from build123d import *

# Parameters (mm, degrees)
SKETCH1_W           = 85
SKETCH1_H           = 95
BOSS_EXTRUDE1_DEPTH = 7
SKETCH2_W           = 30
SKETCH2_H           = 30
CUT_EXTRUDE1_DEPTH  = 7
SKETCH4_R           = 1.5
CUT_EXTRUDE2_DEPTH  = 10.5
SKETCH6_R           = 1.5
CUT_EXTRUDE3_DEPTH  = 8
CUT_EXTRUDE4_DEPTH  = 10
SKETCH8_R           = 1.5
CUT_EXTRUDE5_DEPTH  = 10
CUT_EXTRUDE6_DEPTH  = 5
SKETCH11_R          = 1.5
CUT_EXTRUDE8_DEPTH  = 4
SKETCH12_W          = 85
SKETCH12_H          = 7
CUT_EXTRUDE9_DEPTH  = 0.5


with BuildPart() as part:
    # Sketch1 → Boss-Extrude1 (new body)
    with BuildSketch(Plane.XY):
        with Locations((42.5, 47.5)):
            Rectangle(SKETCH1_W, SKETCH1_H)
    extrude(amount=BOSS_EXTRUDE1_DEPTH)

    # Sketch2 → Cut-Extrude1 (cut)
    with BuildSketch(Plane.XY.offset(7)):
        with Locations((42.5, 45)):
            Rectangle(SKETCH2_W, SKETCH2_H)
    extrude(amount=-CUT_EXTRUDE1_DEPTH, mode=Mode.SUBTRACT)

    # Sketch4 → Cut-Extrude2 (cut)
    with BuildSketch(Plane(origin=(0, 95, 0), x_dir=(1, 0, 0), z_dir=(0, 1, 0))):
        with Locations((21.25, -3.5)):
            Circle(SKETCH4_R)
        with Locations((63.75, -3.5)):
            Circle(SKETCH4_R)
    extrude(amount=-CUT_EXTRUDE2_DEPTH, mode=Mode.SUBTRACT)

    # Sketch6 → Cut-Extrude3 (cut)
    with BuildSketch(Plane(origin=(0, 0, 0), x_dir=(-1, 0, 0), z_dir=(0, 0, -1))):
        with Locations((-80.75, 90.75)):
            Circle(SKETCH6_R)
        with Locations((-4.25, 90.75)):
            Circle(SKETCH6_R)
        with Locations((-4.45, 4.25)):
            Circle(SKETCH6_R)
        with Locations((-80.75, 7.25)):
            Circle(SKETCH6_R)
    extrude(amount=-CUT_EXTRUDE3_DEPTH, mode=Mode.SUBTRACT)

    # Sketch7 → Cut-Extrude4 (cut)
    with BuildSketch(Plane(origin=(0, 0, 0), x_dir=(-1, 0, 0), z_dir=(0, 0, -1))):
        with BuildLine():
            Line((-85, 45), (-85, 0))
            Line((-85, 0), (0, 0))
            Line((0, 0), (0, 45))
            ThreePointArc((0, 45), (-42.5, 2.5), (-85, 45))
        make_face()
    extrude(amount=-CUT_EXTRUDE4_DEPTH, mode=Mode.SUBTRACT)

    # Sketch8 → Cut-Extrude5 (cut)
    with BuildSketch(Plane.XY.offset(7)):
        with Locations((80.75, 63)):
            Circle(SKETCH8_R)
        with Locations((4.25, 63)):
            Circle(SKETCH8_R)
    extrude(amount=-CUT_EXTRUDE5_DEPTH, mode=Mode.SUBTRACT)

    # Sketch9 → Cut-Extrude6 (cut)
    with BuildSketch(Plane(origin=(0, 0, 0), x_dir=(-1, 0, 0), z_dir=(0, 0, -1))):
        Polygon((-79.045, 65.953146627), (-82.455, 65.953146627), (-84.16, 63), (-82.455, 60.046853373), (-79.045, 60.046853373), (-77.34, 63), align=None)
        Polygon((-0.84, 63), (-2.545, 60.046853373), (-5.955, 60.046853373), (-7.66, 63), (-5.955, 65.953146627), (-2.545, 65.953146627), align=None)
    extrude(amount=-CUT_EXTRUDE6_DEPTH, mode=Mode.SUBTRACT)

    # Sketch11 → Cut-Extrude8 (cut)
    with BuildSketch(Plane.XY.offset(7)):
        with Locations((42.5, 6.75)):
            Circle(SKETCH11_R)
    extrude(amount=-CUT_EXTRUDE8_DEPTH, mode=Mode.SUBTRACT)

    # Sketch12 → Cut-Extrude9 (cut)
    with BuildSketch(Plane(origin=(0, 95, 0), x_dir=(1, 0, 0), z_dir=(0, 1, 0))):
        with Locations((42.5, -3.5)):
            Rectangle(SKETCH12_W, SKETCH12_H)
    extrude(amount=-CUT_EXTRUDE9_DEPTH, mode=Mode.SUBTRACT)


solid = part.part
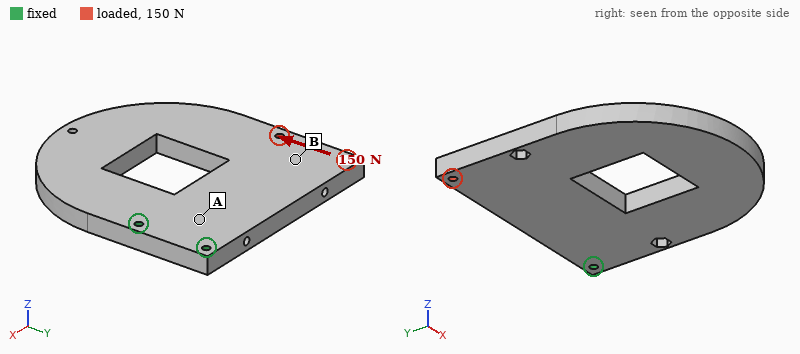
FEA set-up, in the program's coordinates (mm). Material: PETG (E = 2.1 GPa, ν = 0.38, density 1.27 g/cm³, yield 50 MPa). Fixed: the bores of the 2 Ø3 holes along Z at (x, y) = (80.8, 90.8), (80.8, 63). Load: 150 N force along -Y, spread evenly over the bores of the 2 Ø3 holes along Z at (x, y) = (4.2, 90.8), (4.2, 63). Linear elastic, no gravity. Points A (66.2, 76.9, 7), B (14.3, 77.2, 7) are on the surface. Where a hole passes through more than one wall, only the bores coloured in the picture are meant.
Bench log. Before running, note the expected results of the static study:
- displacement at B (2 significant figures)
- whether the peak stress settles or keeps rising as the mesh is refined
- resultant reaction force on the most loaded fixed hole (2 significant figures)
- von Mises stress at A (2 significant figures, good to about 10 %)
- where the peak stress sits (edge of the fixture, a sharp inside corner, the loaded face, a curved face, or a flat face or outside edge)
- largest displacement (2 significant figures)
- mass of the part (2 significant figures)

0.82 mm
keeps rising
410 N
3.7 MPa
edge of the fixture
1.3 mm
54 g
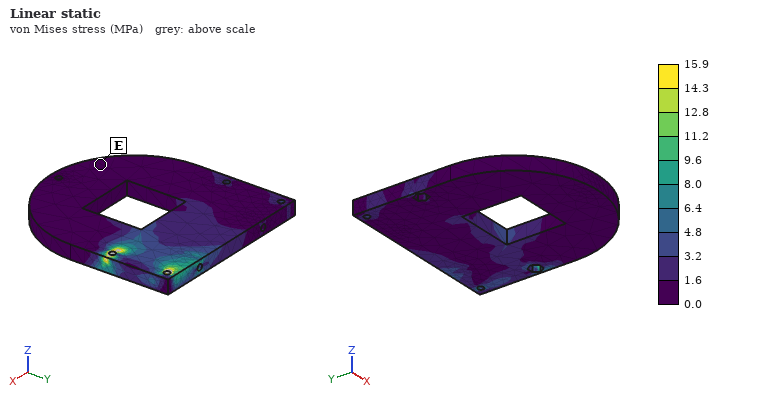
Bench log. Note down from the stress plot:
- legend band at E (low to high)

0.0 to 1.6 MPa
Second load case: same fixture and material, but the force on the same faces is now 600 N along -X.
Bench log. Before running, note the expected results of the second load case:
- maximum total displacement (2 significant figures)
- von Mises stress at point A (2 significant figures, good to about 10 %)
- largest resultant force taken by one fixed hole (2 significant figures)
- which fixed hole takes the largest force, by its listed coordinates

0.42 mm
2.3 MPa
480 N
(80.8, 90.8)
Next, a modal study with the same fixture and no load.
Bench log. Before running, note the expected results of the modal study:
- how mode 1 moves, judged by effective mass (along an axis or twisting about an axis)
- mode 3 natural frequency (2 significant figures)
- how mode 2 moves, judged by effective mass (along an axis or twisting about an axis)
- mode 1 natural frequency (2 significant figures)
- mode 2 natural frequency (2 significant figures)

along Z
510 Hz
twisting about X
120 Hz
280 Hz
